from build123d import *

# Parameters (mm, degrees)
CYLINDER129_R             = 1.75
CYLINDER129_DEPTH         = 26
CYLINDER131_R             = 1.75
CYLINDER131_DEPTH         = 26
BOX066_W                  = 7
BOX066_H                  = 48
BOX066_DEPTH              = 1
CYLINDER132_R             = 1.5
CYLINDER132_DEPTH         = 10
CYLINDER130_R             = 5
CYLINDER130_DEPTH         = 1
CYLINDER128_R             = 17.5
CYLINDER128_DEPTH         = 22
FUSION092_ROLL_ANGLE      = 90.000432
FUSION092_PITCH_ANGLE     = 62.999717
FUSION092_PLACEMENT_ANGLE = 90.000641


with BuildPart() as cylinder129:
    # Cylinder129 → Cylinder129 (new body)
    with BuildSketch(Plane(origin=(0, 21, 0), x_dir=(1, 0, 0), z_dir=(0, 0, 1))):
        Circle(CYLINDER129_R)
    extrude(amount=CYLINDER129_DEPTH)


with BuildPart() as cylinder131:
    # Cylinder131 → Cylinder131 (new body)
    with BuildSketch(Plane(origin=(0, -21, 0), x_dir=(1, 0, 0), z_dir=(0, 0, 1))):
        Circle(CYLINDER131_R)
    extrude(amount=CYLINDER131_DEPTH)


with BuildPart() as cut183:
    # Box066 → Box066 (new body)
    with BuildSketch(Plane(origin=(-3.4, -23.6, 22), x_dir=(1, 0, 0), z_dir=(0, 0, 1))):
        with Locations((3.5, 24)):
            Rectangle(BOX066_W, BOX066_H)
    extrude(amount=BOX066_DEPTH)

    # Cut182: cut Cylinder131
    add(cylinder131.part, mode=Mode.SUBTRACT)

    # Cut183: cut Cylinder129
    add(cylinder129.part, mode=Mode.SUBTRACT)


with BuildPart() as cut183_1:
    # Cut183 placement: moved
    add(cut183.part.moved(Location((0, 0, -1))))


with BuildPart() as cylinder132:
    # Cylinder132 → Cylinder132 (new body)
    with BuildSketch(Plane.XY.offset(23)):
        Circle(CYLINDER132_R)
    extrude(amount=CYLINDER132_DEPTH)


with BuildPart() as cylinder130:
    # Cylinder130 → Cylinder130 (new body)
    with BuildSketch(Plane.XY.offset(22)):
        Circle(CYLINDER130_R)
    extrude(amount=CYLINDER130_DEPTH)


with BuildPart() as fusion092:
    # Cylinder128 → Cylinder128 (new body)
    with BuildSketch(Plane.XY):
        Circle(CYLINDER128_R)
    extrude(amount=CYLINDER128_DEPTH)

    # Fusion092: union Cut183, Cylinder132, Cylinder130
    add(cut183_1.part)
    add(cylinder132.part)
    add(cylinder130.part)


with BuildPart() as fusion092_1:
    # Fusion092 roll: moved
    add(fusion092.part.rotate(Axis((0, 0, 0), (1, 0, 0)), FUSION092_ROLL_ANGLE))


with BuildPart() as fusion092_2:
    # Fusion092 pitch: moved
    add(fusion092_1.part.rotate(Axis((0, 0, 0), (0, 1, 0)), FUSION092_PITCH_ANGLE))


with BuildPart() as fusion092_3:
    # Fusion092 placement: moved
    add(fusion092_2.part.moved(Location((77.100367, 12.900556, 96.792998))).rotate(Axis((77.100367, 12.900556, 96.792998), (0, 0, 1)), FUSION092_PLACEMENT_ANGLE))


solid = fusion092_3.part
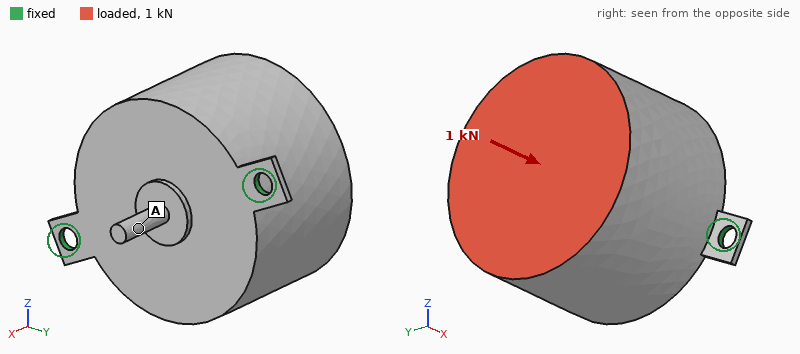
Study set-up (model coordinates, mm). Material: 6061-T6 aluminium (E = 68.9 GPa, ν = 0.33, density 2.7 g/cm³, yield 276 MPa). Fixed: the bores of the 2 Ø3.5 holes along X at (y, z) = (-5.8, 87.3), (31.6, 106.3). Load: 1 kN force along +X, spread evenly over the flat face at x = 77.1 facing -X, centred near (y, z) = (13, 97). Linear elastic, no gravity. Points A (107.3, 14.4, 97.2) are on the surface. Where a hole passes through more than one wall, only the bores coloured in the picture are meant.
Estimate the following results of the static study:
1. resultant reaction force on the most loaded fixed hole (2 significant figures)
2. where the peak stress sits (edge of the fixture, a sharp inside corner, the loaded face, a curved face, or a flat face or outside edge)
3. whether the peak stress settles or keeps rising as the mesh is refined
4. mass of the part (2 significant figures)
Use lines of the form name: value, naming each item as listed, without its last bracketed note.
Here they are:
resultant reaction force on the most loaded fixed hole: 580 N
where the peak stress sits: edge of the fixture
whether the peak stress settles or keeps rising as the mesh is refined: keeps rising
mass of the part: 58 g
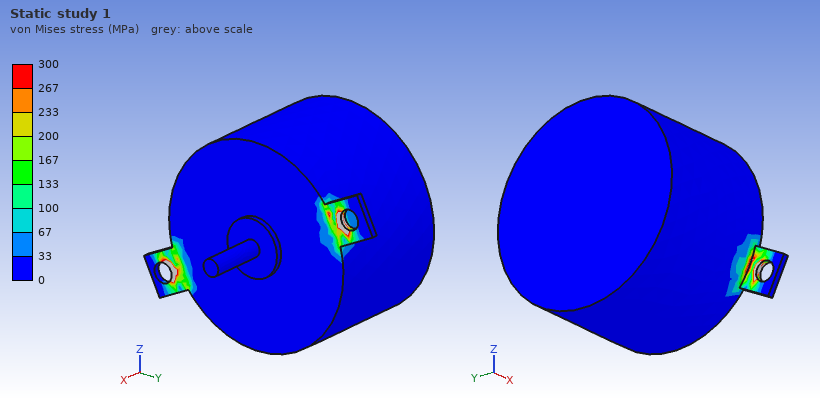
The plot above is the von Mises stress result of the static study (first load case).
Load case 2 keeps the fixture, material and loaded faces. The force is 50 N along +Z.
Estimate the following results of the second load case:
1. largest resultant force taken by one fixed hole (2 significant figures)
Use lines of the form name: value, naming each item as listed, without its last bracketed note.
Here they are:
largest resultant force taken by one fixed hole: 29 N
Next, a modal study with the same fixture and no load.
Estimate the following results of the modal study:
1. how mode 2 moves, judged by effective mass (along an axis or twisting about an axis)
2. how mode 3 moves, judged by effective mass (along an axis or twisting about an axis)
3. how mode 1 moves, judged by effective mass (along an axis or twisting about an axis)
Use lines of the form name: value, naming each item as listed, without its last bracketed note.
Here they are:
how mode 2 moves, judged by effective mass: along X
how mode 3 moves, judged by effective mass: along Y
how mode 1 moves, judged by effective mass: along Z
